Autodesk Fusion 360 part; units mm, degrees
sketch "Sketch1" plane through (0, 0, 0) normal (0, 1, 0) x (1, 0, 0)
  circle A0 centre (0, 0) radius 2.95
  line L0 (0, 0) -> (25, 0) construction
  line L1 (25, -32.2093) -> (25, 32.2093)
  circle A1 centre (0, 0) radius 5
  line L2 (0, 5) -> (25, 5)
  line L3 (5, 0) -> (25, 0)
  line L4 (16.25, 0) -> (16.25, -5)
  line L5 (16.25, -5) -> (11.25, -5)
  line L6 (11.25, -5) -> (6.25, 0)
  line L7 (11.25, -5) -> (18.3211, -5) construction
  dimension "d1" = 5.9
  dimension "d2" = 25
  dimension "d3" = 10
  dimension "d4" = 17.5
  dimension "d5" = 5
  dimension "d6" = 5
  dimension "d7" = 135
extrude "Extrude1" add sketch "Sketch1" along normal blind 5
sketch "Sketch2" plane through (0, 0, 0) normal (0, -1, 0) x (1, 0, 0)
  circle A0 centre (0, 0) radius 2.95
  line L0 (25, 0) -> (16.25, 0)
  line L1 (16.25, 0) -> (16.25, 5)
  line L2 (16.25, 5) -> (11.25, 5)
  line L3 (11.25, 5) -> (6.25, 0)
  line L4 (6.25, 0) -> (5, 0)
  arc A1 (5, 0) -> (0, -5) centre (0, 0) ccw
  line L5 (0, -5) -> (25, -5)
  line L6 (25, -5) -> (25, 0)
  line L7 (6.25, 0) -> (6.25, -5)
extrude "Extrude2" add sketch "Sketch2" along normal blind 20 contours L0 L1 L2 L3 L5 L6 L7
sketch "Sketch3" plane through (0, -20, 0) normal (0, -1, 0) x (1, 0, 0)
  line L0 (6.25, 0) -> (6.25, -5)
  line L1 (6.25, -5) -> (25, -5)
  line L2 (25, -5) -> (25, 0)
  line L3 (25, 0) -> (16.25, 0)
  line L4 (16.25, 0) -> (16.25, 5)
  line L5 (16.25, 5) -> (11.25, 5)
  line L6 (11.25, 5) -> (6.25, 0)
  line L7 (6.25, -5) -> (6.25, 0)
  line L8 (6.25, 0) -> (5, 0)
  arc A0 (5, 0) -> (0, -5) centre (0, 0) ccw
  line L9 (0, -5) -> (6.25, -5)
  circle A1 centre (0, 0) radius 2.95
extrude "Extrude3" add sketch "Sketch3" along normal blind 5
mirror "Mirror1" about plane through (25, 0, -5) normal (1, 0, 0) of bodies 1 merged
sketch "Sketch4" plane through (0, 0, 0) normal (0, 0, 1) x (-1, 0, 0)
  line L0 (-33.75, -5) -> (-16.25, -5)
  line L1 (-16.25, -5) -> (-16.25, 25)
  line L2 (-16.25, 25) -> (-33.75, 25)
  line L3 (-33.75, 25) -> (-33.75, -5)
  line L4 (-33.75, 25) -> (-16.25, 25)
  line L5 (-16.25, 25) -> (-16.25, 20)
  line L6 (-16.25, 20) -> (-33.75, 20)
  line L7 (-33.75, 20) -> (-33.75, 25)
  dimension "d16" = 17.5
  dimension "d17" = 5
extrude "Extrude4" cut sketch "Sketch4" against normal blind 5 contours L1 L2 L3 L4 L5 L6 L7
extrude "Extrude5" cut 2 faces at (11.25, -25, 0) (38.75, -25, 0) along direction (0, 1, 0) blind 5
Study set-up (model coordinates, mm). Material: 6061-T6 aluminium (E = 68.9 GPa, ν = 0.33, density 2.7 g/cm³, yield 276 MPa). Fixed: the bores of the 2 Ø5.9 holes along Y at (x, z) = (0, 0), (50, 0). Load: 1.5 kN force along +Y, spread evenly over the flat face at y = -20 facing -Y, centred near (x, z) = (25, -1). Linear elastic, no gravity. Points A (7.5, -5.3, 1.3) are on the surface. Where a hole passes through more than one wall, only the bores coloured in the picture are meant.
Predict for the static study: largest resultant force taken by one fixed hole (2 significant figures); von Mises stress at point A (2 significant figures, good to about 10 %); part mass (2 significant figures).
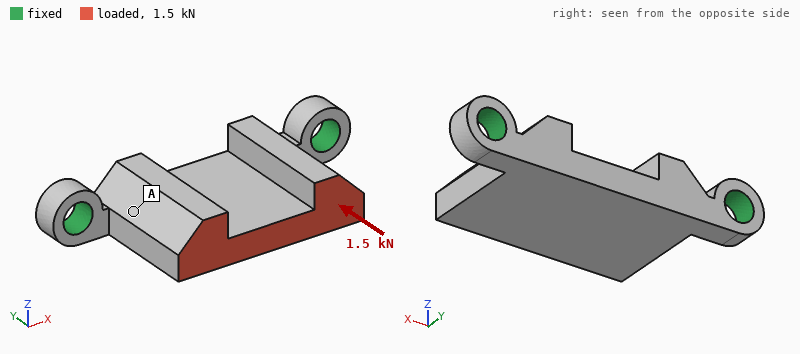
830 N
18 MPa
19 g
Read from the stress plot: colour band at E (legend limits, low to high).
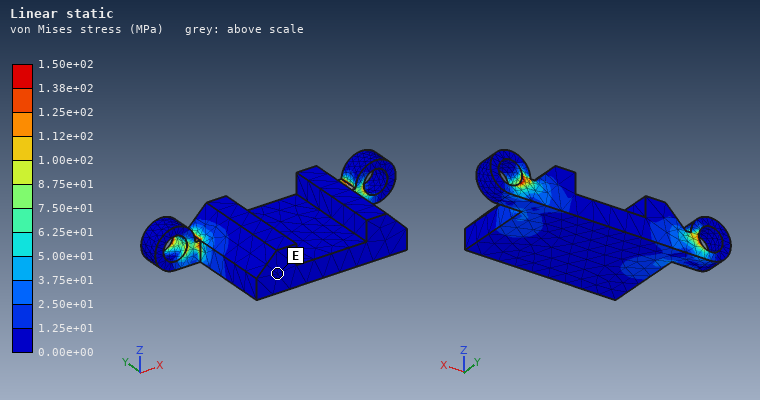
0.00e+00 to 1.25e+01 MPa
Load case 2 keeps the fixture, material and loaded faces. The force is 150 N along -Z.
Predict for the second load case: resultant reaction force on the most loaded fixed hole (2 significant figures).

79 N
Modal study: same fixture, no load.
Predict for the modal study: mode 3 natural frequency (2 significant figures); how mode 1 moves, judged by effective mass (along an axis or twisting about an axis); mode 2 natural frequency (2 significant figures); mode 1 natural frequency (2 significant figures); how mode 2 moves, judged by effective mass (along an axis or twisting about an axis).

11 kHz
along Z
9600 Hz
2800 Hz
twisting about Y
